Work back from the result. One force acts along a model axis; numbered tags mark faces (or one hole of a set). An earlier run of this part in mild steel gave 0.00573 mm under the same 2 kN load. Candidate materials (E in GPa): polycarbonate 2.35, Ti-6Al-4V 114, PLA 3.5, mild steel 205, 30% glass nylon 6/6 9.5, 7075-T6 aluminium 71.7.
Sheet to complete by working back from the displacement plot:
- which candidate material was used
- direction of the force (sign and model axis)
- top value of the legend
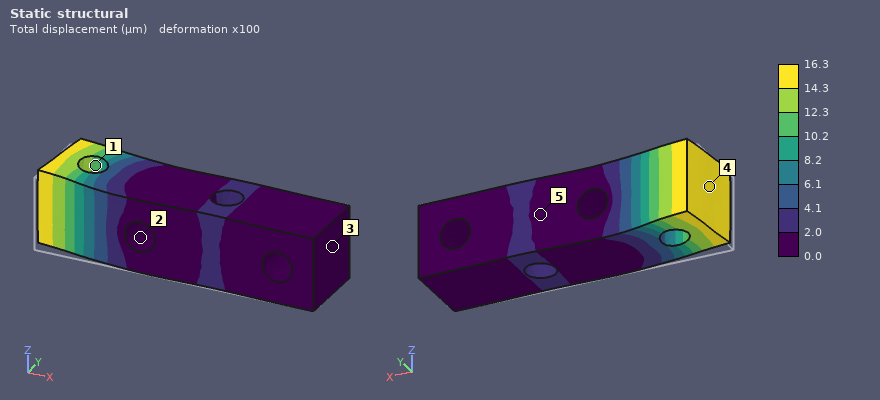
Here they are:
7075-T6 aluminium
+Y
16.3 µm
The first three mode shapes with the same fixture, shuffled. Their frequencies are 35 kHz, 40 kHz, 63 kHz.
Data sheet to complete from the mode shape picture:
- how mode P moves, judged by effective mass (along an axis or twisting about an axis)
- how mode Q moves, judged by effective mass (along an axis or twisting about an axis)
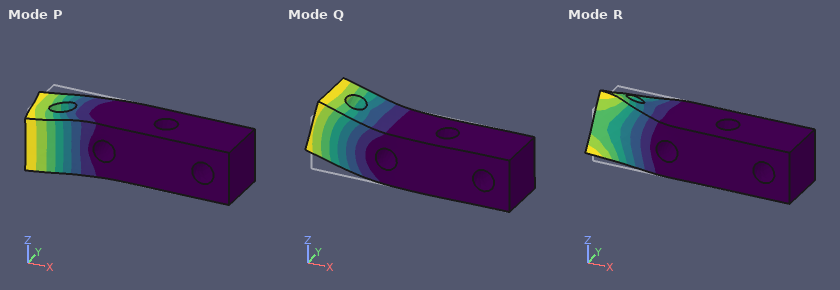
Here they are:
along Y
along Z
